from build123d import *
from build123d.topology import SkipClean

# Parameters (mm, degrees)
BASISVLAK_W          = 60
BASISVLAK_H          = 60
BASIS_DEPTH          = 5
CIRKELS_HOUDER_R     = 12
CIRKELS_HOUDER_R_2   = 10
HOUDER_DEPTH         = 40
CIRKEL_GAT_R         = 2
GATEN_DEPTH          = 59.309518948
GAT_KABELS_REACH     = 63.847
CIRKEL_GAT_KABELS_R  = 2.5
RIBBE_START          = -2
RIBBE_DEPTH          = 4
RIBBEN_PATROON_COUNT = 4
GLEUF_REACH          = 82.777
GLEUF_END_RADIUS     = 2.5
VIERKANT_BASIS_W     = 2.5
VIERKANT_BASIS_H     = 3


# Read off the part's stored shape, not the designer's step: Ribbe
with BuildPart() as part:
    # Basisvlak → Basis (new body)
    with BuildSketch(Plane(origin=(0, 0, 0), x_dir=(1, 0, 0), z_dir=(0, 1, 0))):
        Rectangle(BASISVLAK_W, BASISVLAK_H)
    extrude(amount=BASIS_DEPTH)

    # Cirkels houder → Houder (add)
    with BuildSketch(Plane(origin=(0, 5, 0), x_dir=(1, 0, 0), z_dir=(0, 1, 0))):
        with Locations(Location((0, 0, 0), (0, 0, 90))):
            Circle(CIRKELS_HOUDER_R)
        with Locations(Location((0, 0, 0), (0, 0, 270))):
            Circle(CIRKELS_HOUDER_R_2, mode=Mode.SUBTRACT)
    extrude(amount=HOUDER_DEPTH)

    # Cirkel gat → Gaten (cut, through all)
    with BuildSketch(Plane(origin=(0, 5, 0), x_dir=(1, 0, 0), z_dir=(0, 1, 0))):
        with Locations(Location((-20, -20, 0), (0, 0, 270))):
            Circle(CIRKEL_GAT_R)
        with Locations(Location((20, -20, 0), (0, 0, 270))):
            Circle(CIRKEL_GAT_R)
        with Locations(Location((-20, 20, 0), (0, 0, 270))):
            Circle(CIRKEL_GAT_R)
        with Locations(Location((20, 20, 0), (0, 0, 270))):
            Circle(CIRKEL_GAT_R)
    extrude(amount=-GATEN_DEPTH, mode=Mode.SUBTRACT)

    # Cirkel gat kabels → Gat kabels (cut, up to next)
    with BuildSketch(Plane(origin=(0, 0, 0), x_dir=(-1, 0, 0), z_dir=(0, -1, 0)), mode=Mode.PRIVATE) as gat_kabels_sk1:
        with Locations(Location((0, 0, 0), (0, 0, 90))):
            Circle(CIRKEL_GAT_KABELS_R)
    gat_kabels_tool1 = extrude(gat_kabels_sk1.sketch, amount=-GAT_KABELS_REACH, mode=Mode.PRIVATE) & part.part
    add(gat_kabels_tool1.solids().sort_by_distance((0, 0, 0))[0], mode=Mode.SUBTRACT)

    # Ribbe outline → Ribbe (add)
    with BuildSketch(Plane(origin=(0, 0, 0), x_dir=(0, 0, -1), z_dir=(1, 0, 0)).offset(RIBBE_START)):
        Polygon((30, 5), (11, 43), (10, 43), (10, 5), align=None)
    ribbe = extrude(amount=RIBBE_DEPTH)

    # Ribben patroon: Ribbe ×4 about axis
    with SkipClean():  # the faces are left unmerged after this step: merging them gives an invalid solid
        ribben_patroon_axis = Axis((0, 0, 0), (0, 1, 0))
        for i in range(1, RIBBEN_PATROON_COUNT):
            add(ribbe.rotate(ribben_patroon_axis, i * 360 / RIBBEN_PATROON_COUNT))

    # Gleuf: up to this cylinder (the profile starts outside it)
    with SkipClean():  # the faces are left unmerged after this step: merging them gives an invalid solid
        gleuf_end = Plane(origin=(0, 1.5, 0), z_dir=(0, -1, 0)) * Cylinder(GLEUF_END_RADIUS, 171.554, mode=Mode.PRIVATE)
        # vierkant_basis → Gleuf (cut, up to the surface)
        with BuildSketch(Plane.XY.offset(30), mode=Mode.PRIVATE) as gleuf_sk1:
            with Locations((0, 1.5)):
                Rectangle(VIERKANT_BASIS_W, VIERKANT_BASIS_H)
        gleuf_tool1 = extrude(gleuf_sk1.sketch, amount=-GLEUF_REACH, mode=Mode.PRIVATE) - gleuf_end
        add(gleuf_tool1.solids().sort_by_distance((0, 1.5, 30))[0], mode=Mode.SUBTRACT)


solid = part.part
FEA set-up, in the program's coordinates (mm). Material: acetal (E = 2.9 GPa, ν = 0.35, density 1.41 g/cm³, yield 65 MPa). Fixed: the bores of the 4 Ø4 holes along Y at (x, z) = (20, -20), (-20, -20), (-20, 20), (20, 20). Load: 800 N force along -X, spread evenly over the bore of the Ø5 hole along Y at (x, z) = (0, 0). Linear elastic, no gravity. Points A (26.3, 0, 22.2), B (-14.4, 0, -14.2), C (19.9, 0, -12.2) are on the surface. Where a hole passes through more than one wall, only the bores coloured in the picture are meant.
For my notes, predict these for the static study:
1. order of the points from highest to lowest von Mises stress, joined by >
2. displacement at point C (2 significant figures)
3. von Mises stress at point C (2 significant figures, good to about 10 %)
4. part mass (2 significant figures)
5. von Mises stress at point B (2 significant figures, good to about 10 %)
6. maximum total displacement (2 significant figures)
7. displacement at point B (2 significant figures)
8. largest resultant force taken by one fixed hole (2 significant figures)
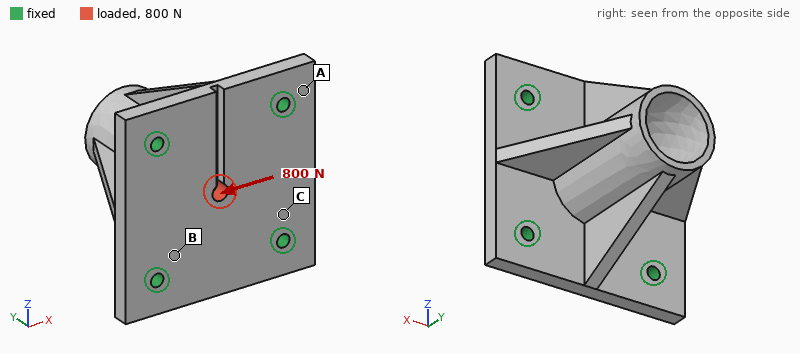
B > C > A
14 µm
2.5 MPa
40 g
3.9 MPa
51 µm
12 µm
230 N
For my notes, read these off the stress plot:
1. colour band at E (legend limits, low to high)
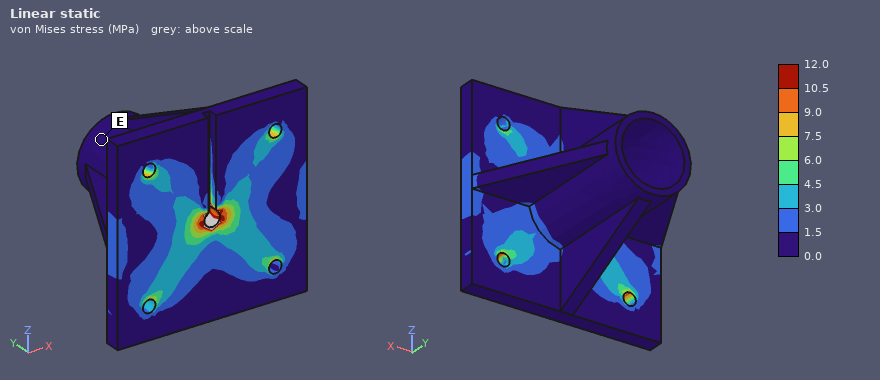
0.0 to 1.5 MPa
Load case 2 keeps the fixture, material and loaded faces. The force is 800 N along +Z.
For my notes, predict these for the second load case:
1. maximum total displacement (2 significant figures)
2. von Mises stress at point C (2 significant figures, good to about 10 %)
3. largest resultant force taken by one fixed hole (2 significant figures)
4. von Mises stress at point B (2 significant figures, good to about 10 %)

51 µm
2.1 MPa
220 N
3.6 MPa
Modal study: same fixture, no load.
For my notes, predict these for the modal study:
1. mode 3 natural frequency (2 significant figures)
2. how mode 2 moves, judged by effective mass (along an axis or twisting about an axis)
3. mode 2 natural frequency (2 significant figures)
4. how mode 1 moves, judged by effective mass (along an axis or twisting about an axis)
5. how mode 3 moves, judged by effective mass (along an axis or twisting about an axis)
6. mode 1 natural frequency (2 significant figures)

2400 Hz
along X
1900 Hz
along Z
along Y
1800 Hz
